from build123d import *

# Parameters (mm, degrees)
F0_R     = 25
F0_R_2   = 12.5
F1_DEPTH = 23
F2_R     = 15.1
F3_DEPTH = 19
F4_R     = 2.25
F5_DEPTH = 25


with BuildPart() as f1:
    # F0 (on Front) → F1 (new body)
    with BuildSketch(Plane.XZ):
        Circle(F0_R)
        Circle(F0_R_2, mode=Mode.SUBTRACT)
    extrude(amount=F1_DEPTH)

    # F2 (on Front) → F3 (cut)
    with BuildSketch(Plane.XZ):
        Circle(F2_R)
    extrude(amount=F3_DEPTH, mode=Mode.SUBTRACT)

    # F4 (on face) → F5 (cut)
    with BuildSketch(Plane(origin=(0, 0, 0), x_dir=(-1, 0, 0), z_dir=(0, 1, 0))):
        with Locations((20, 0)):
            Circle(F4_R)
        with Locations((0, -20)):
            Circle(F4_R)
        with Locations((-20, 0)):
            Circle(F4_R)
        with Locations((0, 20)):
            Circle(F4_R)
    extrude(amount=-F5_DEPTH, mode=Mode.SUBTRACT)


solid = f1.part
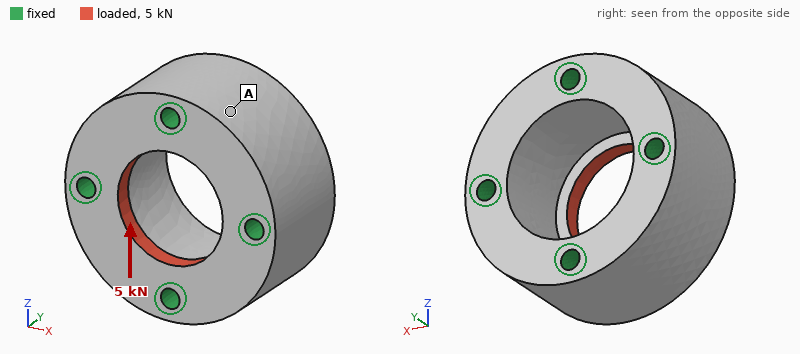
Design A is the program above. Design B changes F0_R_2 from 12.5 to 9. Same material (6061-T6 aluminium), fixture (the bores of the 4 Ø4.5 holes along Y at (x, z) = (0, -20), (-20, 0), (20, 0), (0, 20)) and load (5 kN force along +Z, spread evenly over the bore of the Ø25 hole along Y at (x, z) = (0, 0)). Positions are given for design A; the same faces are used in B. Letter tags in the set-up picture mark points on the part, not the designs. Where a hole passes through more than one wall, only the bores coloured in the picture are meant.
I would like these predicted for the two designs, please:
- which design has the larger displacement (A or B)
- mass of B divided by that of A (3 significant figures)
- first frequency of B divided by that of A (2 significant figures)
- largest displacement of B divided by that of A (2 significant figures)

B
1.03
1.0
1.3
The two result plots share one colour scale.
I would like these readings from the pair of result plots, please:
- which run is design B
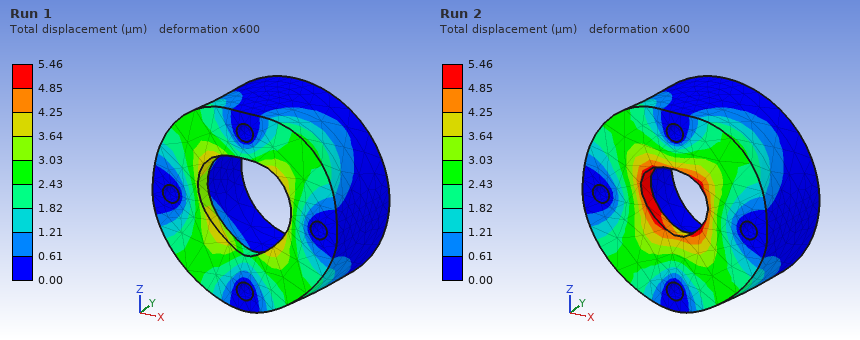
Run 2
